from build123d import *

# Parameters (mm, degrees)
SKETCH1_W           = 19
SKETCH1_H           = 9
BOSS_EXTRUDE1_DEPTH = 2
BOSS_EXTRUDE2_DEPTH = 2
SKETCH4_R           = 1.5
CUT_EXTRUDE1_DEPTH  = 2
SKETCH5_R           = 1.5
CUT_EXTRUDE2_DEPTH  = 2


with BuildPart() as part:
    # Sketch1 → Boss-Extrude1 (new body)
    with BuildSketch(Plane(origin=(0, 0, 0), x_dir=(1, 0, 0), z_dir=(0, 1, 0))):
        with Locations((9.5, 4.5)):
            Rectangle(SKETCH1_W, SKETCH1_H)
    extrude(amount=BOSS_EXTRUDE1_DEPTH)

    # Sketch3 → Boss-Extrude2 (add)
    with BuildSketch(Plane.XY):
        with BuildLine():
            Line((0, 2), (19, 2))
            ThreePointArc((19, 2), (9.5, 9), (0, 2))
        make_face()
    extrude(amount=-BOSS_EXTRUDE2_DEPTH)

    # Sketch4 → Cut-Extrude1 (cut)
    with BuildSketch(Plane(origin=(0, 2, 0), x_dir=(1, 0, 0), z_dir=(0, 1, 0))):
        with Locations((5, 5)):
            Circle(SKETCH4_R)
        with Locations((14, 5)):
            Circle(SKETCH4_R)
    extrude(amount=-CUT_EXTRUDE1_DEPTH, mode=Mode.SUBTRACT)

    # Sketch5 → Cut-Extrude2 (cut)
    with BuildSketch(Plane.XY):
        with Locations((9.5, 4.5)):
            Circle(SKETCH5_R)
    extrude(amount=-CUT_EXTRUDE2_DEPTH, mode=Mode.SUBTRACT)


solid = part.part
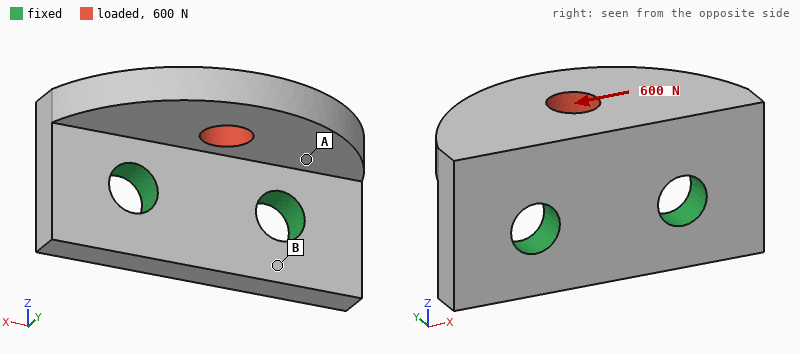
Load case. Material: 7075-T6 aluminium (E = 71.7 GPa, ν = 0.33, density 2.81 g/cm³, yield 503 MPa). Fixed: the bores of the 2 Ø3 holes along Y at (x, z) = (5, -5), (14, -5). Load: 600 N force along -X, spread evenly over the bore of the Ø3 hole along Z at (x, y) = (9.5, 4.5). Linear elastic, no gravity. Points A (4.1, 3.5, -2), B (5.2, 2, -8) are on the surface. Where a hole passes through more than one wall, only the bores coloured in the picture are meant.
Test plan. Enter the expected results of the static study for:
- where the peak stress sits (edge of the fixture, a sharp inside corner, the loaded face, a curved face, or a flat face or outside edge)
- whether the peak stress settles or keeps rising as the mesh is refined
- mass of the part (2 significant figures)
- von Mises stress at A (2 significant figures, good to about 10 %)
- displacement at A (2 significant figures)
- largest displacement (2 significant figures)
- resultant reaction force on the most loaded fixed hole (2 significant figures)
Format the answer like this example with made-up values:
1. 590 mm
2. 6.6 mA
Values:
1. edge of the fixture
2. keeps rising
3. 1.4 g
4. 42 MPa
5. 7.5 µm
6. 14 µm
7. 390 N
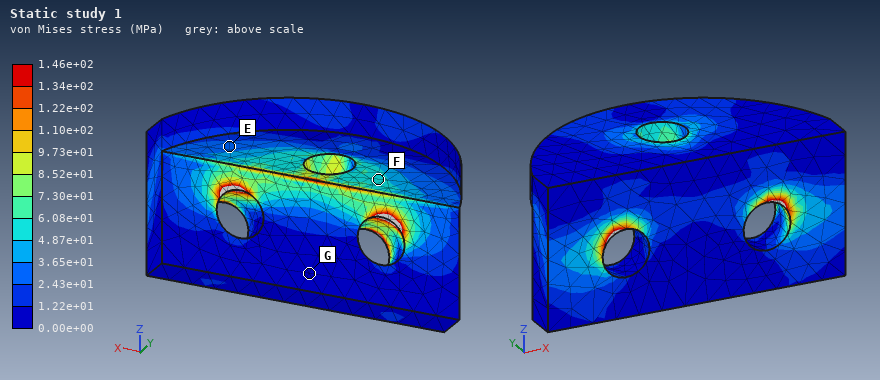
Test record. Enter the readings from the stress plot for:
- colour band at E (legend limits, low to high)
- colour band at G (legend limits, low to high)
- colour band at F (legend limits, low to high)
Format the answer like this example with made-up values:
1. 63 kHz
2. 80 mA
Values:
1. 2.43e+01 to 3.65e+01 MPa
2. 0.00e+00 to 1.22e+01 MPa
3. 4.87e+01 to 6.08e+01 MPa
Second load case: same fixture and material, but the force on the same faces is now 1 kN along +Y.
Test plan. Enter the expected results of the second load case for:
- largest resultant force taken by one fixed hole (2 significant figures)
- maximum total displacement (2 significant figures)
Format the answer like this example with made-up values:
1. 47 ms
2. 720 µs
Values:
1. 510 N
2. 59 µm
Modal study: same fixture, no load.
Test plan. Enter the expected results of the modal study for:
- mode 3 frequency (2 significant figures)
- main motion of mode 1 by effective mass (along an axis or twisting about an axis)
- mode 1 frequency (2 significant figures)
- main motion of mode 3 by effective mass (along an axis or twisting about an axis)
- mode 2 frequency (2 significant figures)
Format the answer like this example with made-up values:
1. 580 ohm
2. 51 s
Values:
1. 54 kHz
2. along Z
3. 21 kHz
4. along X
5. 35 kHz
